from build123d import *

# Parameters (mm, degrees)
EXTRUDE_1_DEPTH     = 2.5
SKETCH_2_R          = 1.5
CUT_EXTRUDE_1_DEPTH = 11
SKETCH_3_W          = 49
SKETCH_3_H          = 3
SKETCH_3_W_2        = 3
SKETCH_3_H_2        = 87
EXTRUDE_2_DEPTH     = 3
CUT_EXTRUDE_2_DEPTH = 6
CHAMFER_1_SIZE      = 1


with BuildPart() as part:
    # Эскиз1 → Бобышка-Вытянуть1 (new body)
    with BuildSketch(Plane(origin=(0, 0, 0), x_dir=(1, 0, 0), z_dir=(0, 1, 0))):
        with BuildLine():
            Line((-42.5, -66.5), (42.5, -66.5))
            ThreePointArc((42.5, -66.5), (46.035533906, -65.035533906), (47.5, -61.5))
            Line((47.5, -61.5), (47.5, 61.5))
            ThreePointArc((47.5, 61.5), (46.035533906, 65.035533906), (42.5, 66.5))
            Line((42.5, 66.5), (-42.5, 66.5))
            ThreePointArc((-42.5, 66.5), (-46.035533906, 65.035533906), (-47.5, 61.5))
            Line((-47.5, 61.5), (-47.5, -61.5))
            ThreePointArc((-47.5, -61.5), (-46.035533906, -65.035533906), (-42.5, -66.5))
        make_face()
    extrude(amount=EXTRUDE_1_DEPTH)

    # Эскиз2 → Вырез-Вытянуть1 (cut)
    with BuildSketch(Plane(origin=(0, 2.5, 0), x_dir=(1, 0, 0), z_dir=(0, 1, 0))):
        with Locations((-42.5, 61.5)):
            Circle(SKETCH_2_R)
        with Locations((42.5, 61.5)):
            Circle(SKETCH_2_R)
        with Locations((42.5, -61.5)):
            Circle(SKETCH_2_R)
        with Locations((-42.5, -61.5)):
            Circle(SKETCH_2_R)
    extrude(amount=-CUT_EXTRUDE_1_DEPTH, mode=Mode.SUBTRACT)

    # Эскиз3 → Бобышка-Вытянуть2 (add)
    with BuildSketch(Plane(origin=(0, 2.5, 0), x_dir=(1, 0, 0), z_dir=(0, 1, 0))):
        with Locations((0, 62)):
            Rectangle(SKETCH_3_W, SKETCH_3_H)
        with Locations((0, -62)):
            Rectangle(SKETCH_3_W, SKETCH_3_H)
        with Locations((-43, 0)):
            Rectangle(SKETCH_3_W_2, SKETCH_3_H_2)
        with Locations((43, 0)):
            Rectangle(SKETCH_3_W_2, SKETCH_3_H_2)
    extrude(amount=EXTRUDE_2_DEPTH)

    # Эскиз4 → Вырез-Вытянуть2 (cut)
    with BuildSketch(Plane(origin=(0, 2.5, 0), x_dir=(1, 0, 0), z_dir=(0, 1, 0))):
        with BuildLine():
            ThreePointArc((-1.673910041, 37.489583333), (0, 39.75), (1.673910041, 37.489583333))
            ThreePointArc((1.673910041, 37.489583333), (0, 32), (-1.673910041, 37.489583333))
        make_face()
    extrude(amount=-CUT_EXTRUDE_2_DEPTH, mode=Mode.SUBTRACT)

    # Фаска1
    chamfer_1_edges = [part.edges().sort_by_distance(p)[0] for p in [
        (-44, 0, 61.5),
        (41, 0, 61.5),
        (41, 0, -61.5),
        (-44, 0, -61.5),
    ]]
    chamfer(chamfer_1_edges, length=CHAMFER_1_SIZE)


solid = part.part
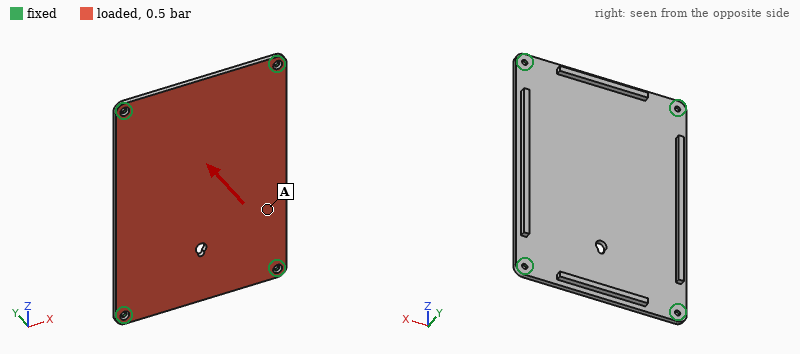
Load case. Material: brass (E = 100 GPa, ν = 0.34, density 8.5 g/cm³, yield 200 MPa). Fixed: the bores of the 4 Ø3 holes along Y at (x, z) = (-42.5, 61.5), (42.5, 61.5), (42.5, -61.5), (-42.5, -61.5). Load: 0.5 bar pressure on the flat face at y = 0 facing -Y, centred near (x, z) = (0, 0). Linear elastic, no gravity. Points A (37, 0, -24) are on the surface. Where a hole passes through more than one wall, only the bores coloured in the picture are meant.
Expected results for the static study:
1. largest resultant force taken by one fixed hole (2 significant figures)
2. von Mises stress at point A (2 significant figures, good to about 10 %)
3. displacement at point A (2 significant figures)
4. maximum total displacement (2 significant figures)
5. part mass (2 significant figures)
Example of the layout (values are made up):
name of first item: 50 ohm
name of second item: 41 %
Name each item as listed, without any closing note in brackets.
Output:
largest resultant force taken by one fixed hole: 160 N
von Mises stress at point A: 21 MPa
displacement at point A: 0.22 mm
maximum total displacement: 0.33 mm
part mass: 290 g
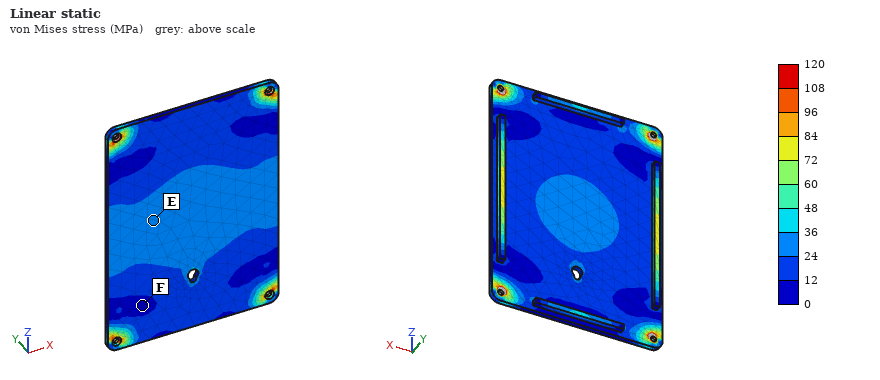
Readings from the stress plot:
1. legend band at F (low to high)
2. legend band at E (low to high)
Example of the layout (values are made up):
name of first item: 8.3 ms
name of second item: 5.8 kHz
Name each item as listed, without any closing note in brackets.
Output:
legend band at F: 0 to 12 MPa
legend band at E: 24 to 36 MPa
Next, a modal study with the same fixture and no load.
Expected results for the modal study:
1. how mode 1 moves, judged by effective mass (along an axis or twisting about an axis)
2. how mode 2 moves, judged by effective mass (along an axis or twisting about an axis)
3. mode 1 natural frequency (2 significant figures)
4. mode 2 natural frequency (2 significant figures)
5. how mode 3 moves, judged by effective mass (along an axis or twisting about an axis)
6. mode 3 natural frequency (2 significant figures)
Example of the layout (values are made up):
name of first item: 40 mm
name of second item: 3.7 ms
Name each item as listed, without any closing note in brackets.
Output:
how mode 1 moves, judged by effective mass: along Y
how mode 2 moves, judged by effective mass: twisting about Z
mode 1 natural frequency: 490 Hz
mode 2 natural frequency: 800 Hz
how mode 3 moves, judged by effective mass: twisting about X
mode 3 natural frequency: 1200 Hz
